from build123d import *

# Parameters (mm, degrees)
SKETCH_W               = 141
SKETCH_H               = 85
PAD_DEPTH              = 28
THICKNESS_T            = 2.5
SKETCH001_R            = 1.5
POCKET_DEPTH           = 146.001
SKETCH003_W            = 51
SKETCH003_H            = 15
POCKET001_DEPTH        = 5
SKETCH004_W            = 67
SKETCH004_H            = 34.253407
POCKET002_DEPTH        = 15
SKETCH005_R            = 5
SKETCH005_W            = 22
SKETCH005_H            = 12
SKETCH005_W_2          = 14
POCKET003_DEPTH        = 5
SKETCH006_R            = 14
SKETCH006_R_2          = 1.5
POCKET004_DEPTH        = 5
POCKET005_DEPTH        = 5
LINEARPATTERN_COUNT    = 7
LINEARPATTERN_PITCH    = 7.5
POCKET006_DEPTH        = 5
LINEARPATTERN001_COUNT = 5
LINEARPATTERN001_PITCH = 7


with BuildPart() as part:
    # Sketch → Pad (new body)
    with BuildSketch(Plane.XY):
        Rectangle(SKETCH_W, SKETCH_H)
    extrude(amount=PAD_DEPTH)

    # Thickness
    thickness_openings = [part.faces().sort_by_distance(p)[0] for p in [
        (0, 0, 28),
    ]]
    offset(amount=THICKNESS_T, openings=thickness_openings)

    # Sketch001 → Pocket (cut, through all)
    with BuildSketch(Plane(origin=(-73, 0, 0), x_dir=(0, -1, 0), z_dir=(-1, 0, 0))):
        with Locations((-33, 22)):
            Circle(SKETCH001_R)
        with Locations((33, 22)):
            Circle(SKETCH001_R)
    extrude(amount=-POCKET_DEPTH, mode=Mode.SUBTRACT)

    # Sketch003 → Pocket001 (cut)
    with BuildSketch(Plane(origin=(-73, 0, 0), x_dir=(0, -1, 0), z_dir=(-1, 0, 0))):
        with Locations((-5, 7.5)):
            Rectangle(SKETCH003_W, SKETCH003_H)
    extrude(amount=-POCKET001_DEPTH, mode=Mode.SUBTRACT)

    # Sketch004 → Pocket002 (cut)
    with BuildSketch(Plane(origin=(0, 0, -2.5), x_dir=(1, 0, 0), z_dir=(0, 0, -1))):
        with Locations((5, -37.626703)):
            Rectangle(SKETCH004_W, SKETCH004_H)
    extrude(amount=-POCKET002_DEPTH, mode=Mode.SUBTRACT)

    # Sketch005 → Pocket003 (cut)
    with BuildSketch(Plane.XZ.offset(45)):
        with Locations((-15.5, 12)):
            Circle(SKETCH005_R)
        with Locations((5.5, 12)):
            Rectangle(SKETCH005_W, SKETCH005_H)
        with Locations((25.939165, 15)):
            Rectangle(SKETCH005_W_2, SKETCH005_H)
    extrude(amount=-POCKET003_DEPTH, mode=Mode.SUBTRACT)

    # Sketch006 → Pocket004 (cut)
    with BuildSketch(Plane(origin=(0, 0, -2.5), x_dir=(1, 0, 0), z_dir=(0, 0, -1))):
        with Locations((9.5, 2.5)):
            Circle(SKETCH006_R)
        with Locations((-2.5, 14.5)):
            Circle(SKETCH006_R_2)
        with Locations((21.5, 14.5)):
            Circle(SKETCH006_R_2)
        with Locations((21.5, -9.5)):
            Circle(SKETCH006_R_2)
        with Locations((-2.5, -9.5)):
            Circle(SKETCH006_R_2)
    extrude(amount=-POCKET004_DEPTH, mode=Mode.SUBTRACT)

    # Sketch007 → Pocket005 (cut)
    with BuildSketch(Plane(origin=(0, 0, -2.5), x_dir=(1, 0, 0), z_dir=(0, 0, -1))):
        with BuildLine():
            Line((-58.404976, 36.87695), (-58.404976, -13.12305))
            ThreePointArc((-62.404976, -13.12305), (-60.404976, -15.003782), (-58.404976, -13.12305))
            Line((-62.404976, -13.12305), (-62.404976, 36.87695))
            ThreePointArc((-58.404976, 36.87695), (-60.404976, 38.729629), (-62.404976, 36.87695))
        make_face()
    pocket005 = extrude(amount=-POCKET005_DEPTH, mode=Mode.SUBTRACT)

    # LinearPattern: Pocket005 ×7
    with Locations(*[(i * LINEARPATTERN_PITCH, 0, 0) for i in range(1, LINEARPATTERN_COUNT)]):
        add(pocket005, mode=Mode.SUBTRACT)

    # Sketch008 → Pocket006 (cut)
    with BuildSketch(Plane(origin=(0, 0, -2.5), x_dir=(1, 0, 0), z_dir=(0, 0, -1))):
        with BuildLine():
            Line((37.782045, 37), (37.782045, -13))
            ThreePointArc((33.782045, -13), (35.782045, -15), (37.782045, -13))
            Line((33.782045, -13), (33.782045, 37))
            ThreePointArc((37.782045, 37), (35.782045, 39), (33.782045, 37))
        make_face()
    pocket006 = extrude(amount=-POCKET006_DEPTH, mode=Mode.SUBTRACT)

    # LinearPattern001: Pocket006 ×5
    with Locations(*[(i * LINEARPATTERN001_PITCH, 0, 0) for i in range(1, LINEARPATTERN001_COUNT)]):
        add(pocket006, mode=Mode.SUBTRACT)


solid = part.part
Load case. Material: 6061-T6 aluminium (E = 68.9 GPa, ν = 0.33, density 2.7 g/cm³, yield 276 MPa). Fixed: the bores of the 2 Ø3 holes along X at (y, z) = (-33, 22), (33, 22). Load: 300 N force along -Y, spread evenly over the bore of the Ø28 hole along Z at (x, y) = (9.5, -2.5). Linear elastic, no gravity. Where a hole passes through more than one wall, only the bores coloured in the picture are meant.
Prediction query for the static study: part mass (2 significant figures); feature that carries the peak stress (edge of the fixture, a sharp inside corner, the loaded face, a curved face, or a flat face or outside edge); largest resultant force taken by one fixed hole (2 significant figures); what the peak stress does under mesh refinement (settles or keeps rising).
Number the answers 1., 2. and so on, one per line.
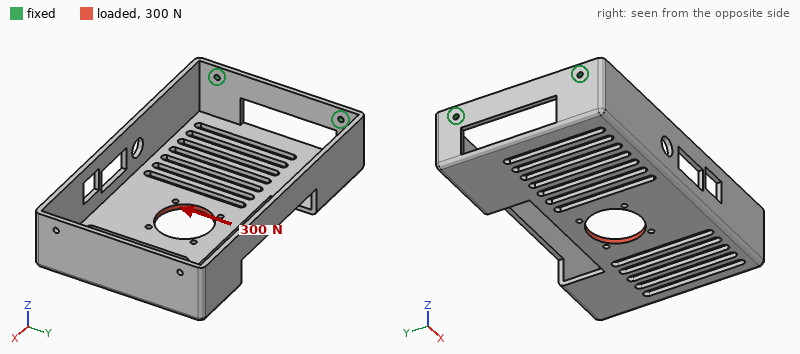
1. 130 g
2. edge of the fixture
3. 360 N
4. keeps rising
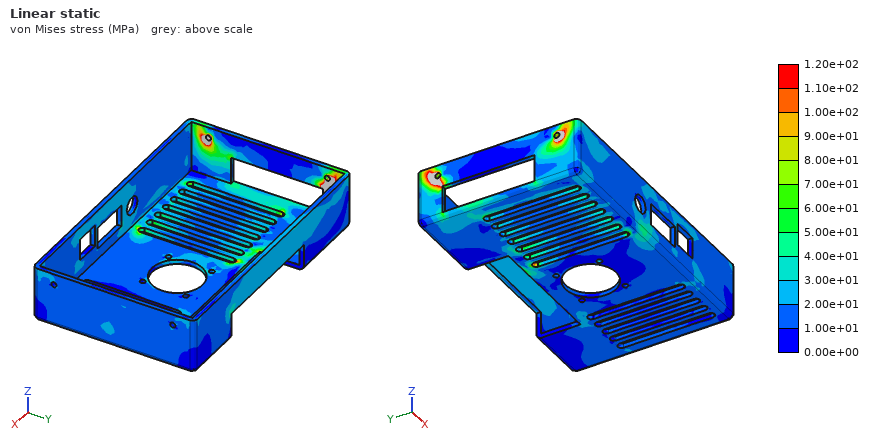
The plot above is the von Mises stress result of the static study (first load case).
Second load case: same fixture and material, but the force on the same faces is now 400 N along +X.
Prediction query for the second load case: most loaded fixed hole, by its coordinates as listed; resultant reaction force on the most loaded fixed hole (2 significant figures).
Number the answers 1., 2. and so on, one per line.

1. (-33, 22)
2. 220 N
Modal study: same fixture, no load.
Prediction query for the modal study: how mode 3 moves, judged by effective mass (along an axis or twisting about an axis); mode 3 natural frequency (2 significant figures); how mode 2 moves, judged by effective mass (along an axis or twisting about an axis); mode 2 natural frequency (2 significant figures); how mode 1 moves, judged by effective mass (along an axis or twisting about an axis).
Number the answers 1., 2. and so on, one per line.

1. along Y
2. 690 Hz
3. along Y
4. 190 Hz
5. along Z
